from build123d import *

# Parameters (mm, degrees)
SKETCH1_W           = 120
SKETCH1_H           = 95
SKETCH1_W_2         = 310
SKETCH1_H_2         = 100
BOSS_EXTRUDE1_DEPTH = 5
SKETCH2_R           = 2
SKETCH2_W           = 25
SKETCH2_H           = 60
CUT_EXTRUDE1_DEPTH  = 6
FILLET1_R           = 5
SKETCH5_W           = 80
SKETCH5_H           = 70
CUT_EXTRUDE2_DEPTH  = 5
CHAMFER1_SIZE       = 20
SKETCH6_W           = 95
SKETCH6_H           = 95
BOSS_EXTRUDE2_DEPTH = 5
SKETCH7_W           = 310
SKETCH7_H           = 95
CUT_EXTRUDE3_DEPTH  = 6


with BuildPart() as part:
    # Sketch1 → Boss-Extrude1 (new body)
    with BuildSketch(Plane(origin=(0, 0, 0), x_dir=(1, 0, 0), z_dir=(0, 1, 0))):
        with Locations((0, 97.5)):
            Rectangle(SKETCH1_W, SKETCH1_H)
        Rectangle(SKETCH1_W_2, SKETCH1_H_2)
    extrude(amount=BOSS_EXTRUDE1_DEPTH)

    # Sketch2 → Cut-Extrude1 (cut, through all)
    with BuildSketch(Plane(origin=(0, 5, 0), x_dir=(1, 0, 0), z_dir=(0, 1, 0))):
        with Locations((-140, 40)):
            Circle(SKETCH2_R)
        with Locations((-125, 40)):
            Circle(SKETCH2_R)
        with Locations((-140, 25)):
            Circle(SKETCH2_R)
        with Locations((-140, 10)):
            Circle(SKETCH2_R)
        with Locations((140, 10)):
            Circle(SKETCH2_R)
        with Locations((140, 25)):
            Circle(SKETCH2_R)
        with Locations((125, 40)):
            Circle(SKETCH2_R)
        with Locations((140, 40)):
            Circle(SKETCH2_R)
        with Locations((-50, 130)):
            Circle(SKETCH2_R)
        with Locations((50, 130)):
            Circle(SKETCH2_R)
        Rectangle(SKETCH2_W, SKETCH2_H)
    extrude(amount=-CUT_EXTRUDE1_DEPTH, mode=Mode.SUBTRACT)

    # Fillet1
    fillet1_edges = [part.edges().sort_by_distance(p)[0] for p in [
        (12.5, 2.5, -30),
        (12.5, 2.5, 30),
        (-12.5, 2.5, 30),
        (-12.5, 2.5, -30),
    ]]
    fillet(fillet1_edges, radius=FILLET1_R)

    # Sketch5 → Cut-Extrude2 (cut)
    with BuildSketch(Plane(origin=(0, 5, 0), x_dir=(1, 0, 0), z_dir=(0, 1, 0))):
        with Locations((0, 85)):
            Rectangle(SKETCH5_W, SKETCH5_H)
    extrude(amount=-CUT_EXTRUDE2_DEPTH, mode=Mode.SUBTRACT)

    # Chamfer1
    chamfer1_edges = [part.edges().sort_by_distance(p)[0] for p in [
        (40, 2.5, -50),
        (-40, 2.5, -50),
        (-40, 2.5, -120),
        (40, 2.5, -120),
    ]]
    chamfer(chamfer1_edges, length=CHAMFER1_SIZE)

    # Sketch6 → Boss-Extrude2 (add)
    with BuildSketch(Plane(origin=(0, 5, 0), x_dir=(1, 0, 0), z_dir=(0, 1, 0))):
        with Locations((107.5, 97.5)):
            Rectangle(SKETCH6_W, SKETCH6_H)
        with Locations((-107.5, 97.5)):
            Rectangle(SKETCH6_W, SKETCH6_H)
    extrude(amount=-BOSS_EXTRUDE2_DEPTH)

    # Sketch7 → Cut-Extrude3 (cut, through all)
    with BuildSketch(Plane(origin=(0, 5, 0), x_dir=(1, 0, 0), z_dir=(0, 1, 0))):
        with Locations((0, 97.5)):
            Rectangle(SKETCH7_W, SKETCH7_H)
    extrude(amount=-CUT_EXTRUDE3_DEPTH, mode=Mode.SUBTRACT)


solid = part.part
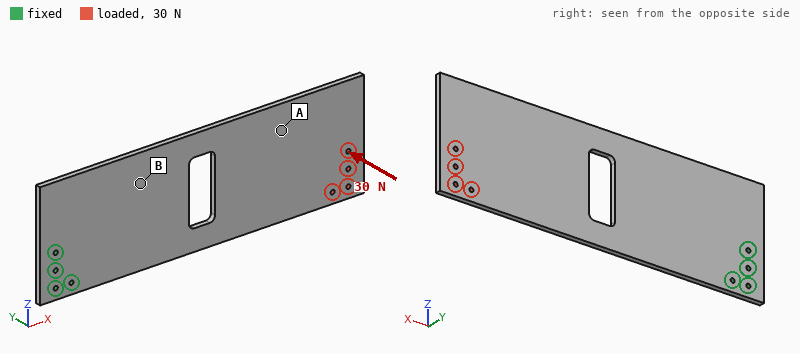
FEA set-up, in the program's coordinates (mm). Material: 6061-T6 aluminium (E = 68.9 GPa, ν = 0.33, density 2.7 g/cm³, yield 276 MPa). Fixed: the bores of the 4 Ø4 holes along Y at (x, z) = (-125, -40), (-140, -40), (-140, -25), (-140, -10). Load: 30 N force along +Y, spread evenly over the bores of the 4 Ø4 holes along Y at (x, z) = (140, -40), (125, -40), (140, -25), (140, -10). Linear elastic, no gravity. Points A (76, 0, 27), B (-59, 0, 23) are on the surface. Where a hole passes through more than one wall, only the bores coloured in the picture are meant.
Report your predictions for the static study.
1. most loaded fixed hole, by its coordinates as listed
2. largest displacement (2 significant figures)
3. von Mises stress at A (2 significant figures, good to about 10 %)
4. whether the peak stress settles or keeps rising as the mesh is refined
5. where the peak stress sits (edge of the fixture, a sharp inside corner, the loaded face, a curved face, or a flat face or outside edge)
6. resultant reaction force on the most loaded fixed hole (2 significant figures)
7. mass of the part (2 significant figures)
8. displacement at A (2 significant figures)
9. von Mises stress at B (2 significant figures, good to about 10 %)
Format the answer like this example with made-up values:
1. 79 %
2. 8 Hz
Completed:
1. (-125, -40)
2. 3.9 mm
3. 4.6 MPa
4. keeps rising
5. edge of the fixture
6. 180 N
7. 400 g
8. 2.2 mm
9. 13 MPa
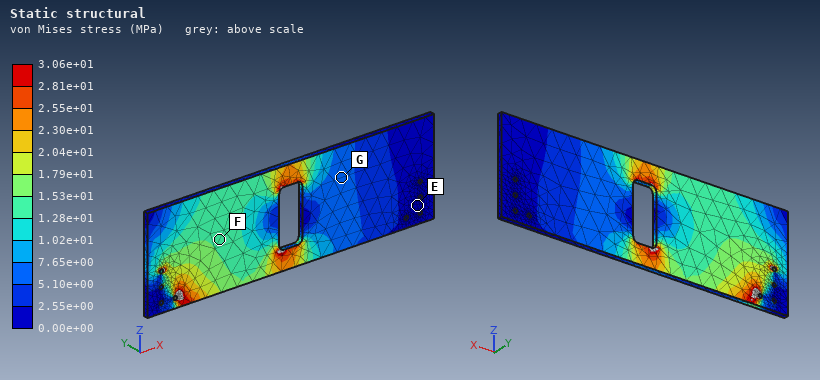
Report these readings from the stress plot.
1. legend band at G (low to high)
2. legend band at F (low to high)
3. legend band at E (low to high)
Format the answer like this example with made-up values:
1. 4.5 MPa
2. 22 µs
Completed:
1. 5.10e+00 to 7.65e+00 MPa
2. 1.28e+01 to 1.53e+01 MPa
3. 0.00e+00 to 2.55e+00 MPa
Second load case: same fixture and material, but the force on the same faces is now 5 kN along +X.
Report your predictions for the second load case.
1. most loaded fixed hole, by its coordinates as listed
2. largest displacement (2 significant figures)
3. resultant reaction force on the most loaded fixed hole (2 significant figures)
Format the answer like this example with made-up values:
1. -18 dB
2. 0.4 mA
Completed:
1. (-125, -40)
2. 0.23 mm
3. 2.1 kN
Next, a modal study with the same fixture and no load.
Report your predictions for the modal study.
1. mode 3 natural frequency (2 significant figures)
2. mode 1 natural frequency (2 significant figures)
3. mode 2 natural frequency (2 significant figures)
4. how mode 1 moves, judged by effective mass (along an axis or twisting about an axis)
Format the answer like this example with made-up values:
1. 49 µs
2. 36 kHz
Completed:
1. 280 Hz
2. 45 Hz
3. 240 Hz
4. along Y
